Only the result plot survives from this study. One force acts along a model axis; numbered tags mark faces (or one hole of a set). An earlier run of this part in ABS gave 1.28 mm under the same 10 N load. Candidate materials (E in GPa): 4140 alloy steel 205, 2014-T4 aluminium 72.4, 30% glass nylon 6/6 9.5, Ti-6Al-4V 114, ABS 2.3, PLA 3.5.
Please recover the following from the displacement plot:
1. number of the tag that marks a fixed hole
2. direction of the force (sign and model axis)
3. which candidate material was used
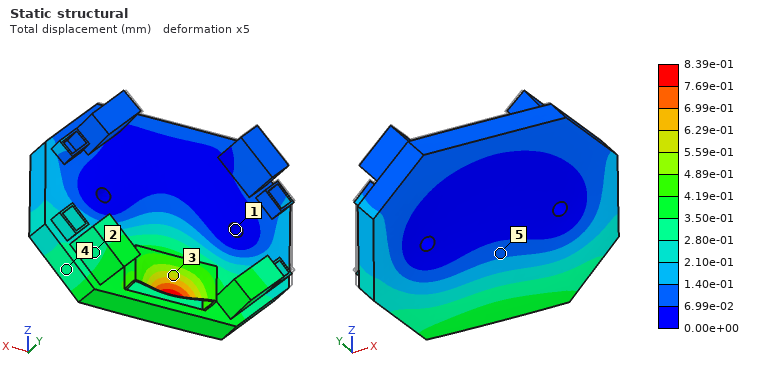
1
-Y
PLA
